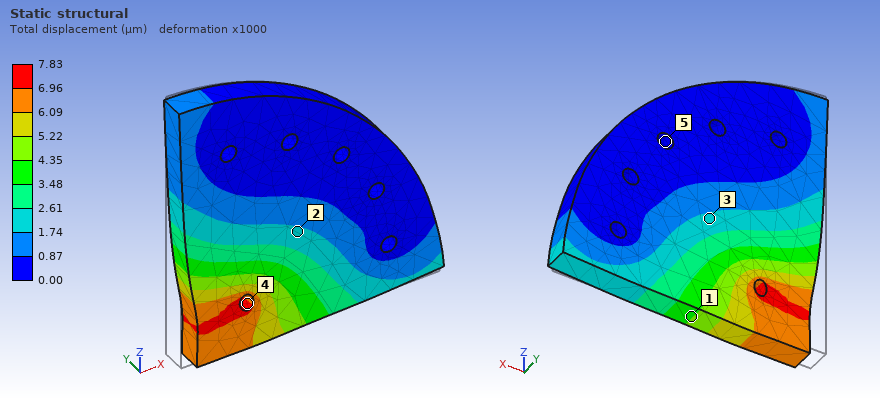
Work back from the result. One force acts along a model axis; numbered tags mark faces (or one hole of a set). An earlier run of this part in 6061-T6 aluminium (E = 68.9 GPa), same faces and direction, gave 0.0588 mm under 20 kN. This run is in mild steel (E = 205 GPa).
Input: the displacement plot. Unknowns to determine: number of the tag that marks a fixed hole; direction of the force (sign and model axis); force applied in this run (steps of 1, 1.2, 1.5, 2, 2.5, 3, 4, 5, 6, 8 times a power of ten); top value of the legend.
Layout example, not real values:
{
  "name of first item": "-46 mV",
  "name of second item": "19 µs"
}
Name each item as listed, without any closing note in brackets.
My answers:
{
  "number of the tag that marks a fixed hole": "5",
  "direction of the force": "+X",
  "force applied in this run": "8 kN",
  "top value of the legend": "7.83 µm"
}
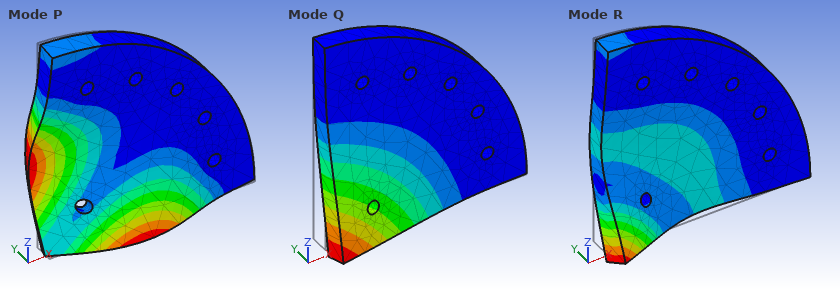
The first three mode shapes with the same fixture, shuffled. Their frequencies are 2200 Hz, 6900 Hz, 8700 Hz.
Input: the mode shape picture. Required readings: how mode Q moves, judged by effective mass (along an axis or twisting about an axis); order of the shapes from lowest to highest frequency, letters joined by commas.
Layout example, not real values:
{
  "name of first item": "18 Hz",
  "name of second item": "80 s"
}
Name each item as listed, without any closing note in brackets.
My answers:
{
  "how mode Q moves, judged by effective mass": "along Y",
  "order of the shapes from lowest to highest frequency, letters joined by commas": "Q, P, R"
}
